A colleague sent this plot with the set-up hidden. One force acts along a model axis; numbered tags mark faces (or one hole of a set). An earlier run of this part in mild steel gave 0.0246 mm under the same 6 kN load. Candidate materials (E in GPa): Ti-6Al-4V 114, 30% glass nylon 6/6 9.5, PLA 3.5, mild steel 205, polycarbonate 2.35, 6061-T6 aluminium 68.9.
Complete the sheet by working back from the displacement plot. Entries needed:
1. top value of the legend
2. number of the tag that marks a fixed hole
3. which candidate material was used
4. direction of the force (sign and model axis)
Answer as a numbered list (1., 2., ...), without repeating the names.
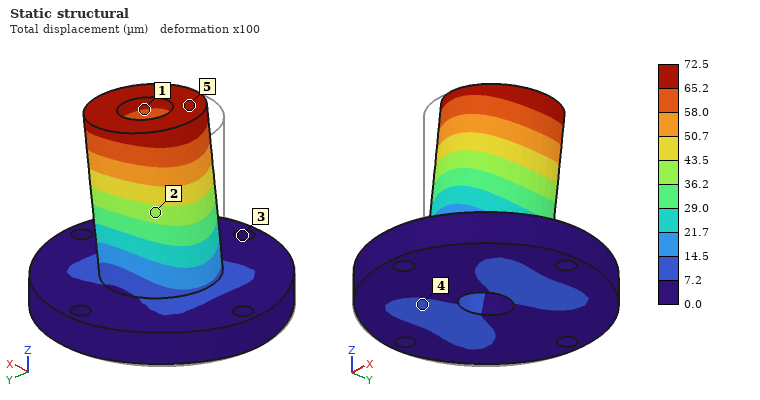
1. 72.5 µm
2. 3
3. 6061-T6 aluminium
4. +X
